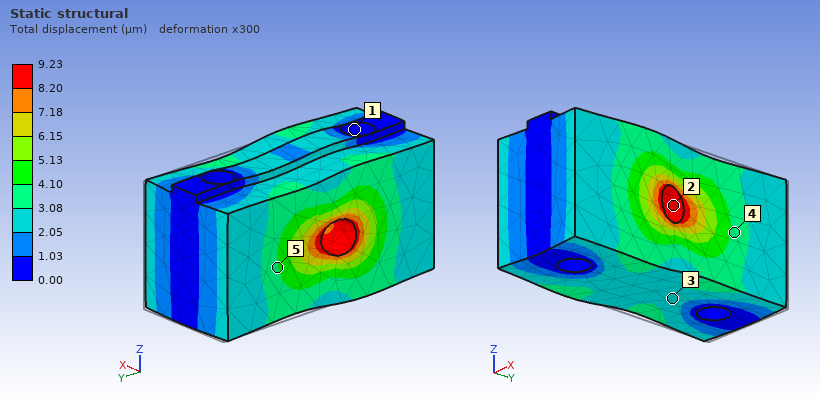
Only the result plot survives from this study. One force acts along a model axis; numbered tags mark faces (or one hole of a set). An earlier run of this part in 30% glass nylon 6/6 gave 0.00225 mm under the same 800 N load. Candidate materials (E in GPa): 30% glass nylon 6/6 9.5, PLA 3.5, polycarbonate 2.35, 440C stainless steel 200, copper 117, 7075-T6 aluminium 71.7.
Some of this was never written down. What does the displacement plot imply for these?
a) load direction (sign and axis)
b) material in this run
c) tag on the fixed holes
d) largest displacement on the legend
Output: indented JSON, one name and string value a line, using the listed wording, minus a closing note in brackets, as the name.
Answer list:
{
  "load direction": "-Y",
  "material in this run": "polycarbonate",
  "tag on the fixed holes": "1",
  "largest displacement on the legend": "9.23 µm"
}
